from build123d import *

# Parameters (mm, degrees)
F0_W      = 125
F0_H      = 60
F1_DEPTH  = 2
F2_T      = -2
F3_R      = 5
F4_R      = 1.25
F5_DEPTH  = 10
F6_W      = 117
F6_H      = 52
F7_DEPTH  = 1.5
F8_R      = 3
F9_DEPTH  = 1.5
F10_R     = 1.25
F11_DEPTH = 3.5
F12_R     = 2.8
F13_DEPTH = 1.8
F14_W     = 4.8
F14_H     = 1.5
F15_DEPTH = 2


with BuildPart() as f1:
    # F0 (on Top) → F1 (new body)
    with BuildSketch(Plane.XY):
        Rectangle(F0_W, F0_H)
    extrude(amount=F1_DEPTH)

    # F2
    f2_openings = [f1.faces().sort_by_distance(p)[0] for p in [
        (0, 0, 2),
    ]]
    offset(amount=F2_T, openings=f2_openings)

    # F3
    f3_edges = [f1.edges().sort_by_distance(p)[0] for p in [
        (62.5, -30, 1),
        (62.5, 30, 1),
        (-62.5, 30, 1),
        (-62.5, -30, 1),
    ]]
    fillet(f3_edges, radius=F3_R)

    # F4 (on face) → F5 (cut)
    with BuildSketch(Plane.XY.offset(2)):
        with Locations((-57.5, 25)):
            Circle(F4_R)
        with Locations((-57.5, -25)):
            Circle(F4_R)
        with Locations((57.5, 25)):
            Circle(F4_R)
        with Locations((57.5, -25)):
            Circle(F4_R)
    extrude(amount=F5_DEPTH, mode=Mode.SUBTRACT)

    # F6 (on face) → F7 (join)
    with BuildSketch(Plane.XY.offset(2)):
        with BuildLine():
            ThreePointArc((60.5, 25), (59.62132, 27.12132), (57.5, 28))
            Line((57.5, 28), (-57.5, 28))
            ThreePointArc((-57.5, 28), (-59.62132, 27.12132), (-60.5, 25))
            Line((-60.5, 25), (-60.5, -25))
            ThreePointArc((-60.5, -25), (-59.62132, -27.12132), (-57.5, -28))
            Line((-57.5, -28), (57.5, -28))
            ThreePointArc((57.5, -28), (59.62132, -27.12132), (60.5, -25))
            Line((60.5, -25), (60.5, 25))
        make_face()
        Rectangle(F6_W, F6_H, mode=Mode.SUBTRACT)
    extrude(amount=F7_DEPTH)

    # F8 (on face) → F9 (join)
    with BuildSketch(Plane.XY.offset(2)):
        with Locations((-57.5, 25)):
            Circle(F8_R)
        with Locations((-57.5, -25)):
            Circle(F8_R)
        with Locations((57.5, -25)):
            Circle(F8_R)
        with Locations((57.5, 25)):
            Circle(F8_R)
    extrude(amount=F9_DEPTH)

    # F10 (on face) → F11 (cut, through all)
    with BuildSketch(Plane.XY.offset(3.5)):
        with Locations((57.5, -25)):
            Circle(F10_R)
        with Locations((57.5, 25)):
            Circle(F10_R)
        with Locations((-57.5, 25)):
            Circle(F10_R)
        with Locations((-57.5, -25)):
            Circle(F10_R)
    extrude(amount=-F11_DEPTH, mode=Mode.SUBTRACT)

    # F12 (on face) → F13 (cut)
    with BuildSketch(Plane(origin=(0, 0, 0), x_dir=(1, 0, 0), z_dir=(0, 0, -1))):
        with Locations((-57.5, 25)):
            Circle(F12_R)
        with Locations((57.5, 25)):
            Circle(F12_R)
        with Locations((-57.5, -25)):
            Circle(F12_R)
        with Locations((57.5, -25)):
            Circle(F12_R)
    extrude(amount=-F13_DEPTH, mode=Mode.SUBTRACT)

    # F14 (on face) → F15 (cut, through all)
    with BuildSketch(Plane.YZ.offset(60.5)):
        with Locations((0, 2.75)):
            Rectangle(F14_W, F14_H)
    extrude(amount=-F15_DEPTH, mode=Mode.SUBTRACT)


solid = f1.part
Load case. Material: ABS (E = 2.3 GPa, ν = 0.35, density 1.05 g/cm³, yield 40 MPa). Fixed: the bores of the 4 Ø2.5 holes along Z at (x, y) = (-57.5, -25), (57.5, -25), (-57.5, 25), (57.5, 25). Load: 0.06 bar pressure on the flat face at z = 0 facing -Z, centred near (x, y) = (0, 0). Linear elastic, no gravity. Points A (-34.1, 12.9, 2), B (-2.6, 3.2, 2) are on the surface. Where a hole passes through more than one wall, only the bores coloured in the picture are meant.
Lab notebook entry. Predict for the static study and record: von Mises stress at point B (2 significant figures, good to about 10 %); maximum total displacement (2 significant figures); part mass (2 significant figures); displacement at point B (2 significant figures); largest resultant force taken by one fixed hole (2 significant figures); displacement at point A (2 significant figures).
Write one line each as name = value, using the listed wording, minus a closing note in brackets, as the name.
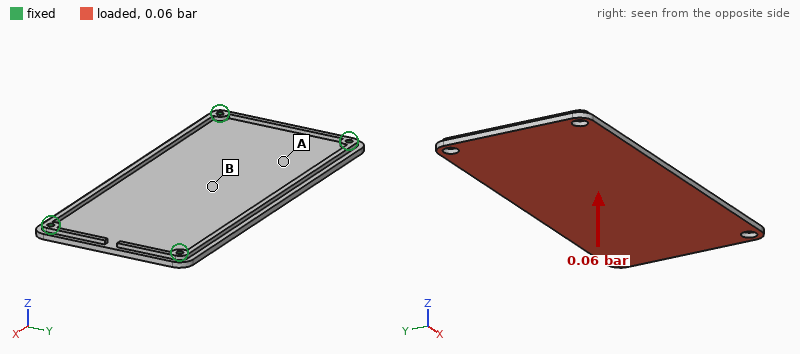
von Mises stress at point B = 3.0 MPa
maximum total displacement = 1.7 mm
part mass = 17 g
displacement at point B = 1.6 mm
largest resultant force taken by one fixed hole = 42 N
displacement at point A = 0.84 mm
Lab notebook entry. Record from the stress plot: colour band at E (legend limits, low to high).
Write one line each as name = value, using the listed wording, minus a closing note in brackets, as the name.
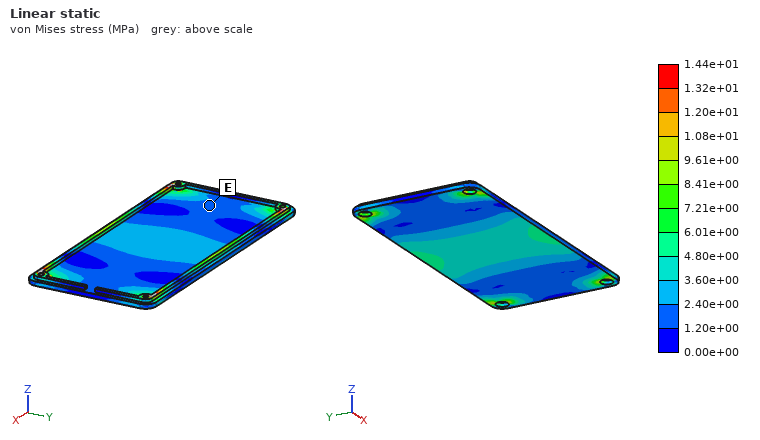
colour band at E = 1.20e+00 to 2.40e+00 MPa
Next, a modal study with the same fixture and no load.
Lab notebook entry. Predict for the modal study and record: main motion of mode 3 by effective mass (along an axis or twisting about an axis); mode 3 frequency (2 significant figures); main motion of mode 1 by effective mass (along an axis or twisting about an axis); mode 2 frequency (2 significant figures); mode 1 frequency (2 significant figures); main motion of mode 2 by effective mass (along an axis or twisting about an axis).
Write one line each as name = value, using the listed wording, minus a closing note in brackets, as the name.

main motion of mode 3 by effective mass = twisting about Y
mode 3 frequency = 620 Hz
main motion of mode 1 by effective mass = along Z
mode 2 frequency = 400 Hz
mode 1 frequency = 230 Hz
main motion of mode 2 by effective mass = twisting about X
